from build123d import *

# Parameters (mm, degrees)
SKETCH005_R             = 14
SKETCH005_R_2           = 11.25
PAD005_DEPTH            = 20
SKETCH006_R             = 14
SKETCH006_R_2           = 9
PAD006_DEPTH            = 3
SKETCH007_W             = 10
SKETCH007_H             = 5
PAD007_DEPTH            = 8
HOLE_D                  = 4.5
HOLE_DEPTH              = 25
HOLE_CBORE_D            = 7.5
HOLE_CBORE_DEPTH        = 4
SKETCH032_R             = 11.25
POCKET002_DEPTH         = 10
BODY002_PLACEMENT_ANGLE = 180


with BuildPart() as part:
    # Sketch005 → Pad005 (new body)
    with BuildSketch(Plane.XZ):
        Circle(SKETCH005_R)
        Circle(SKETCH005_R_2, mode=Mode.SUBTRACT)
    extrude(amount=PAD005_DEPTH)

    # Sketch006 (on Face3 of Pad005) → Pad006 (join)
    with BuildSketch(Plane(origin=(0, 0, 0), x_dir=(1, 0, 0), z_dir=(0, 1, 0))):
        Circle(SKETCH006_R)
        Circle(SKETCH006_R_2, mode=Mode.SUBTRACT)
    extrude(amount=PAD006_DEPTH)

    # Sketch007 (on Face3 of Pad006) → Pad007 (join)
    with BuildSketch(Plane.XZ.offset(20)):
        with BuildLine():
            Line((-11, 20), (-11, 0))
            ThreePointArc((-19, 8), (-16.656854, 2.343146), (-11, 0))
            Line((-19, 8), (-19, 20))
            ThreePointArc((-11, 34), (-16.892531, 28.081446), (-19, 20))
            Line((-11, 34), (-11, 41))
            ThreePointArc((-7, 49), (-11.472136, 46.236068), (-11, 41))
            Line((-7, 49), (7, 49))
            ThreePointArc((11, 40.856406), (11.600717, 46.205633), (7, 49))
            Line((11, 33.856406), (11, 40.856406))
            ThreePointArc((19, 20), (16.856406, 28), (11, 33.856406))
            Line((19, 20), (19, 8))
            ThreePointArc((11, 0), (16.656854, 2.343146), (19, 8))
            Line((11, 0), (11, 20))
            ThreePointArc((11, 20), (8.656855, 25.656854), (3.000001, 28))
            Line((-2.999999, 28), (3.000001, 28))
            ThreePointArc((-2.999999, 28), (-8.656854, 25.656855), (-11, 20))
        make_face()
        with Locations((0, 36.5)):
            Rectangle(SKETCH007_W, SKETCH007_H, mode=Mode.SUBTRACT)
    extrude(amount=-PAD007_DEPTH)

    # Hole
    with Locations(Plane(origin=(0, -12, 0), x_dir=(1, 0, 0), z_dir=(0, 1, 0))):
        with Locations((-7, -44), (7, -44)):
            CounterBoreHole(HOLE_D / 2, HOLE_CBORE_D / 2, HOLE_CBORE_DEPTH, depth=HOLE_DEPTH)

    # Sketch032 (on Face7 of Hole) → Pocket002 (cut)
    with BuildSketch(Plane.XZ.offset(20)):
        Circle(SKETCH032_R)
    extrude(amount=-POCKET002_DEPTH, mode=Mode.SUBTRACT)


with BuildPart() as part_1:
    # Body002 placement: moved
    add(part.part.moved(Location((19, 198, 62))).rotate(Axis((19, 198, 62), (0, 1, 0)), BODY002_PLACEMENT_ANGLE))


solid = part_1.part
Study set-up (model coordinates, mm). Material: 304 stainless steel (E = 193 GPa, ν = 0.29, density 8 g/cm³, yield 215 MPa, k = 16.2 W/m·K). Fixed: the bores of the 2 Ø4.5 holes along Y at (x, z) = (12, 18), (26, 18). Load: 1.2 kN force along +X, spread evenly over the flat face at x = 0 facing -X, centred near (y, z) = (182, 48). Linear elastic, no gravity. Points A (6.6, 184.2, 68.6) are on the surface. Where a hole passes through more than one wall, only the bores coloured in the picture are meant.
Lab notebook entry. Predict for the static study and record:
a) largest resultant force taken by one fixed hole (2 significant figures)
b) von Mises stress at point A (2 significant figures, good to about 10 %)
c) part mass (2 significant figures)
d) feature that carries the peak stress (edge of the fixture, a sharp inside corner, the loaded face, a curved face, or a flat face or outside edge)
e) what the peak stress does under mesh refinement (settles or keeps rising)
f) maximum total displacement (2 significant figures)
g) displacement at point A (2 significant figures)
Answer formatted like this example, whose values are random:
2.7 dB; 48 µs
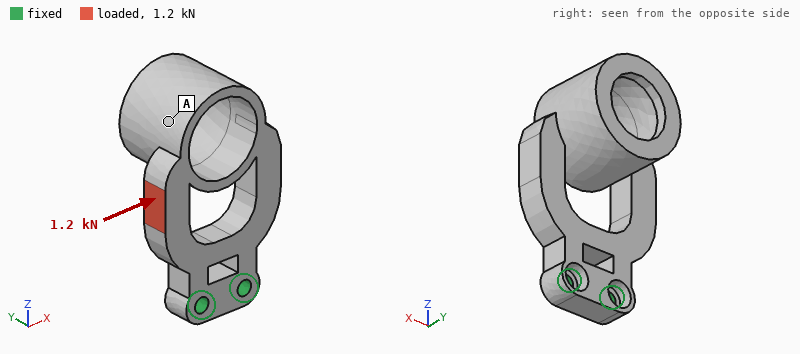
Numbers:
2.0 kN; 17 MPa; 95 g; edge of the fixture; keeps rising; 89 µm; 81 µm
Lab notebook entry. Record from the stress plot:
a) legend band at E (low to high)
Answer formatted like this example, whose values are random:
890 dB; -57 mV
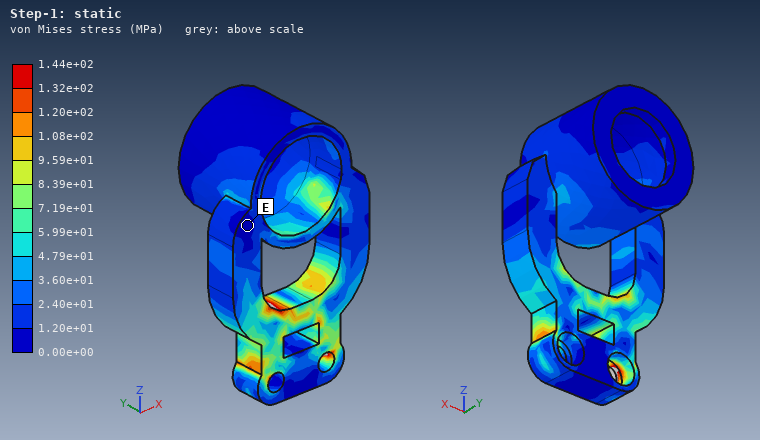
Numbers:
0.00e+00 to 1.20e+01 MPa
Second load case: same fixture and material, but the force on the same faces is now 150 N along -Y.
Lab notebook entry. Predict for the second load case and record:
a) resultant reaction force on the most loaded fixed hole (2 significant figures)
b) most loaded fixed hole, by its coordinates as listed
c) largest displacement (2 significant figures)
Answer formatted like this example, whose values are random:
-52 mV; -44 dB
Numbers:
250 N; (12, 18); 52 µm
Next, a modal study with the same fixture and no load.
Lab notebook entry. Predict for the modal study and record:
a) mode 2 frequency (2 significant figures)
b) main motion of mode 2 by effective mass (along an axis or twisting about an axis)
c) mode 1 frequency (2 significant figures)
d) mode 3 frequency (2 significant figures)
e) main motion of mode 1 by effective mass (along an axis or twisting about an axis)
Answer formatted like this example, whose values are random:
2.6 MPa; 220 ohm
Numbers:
2100 Hz; along X; 1000 Hz; 3200 Hz; along Y
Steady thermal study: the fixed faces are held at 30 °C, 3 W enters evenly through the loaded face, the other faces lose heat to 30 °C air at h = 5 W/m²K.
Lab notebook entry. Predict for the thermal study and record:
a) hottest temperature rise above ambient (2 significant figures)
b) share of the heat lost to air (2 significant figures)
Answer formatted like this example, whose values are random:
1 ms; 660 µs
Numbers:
53 K; 31 %
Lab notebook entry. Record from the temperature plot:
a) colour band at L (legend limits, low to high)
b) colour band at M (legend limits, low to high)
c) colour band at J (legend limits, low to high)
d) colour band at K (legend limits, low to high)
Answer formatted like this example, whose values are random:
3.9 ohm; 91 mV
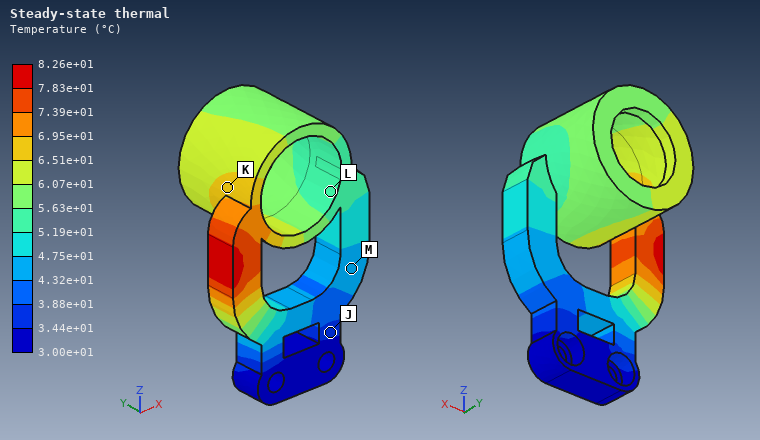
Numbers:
5.19e+01 to 5.63e+01 °C; 4.32e+01 to 4.75e+01 °C; 3.44e+01 to 3.88e+01 °C; 6.51e+01 to 6.95e+01 °C
